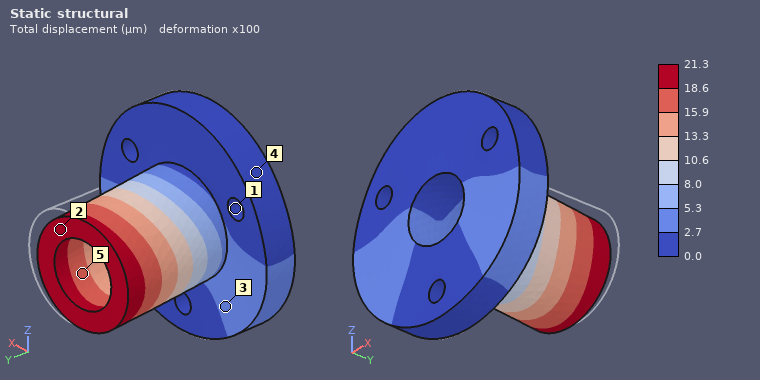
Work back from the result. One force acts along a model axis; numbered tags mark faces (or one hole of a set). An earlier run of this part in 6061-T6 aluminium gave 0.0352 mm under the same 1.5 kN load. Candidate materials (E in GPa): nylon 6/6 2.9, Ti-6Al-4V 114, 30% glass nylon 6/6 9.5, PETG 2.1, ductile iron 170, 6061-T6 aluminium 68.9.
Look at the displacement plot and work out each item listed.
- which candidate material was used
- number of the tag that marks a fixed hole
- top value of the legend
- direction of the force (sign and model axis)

Ti-6Al-4V
1
21.3 µm
-X
